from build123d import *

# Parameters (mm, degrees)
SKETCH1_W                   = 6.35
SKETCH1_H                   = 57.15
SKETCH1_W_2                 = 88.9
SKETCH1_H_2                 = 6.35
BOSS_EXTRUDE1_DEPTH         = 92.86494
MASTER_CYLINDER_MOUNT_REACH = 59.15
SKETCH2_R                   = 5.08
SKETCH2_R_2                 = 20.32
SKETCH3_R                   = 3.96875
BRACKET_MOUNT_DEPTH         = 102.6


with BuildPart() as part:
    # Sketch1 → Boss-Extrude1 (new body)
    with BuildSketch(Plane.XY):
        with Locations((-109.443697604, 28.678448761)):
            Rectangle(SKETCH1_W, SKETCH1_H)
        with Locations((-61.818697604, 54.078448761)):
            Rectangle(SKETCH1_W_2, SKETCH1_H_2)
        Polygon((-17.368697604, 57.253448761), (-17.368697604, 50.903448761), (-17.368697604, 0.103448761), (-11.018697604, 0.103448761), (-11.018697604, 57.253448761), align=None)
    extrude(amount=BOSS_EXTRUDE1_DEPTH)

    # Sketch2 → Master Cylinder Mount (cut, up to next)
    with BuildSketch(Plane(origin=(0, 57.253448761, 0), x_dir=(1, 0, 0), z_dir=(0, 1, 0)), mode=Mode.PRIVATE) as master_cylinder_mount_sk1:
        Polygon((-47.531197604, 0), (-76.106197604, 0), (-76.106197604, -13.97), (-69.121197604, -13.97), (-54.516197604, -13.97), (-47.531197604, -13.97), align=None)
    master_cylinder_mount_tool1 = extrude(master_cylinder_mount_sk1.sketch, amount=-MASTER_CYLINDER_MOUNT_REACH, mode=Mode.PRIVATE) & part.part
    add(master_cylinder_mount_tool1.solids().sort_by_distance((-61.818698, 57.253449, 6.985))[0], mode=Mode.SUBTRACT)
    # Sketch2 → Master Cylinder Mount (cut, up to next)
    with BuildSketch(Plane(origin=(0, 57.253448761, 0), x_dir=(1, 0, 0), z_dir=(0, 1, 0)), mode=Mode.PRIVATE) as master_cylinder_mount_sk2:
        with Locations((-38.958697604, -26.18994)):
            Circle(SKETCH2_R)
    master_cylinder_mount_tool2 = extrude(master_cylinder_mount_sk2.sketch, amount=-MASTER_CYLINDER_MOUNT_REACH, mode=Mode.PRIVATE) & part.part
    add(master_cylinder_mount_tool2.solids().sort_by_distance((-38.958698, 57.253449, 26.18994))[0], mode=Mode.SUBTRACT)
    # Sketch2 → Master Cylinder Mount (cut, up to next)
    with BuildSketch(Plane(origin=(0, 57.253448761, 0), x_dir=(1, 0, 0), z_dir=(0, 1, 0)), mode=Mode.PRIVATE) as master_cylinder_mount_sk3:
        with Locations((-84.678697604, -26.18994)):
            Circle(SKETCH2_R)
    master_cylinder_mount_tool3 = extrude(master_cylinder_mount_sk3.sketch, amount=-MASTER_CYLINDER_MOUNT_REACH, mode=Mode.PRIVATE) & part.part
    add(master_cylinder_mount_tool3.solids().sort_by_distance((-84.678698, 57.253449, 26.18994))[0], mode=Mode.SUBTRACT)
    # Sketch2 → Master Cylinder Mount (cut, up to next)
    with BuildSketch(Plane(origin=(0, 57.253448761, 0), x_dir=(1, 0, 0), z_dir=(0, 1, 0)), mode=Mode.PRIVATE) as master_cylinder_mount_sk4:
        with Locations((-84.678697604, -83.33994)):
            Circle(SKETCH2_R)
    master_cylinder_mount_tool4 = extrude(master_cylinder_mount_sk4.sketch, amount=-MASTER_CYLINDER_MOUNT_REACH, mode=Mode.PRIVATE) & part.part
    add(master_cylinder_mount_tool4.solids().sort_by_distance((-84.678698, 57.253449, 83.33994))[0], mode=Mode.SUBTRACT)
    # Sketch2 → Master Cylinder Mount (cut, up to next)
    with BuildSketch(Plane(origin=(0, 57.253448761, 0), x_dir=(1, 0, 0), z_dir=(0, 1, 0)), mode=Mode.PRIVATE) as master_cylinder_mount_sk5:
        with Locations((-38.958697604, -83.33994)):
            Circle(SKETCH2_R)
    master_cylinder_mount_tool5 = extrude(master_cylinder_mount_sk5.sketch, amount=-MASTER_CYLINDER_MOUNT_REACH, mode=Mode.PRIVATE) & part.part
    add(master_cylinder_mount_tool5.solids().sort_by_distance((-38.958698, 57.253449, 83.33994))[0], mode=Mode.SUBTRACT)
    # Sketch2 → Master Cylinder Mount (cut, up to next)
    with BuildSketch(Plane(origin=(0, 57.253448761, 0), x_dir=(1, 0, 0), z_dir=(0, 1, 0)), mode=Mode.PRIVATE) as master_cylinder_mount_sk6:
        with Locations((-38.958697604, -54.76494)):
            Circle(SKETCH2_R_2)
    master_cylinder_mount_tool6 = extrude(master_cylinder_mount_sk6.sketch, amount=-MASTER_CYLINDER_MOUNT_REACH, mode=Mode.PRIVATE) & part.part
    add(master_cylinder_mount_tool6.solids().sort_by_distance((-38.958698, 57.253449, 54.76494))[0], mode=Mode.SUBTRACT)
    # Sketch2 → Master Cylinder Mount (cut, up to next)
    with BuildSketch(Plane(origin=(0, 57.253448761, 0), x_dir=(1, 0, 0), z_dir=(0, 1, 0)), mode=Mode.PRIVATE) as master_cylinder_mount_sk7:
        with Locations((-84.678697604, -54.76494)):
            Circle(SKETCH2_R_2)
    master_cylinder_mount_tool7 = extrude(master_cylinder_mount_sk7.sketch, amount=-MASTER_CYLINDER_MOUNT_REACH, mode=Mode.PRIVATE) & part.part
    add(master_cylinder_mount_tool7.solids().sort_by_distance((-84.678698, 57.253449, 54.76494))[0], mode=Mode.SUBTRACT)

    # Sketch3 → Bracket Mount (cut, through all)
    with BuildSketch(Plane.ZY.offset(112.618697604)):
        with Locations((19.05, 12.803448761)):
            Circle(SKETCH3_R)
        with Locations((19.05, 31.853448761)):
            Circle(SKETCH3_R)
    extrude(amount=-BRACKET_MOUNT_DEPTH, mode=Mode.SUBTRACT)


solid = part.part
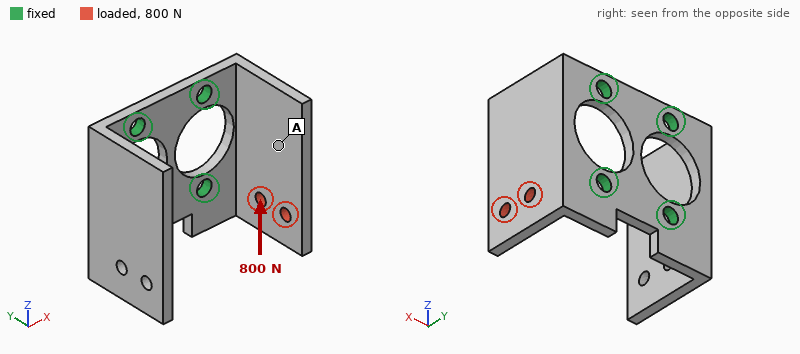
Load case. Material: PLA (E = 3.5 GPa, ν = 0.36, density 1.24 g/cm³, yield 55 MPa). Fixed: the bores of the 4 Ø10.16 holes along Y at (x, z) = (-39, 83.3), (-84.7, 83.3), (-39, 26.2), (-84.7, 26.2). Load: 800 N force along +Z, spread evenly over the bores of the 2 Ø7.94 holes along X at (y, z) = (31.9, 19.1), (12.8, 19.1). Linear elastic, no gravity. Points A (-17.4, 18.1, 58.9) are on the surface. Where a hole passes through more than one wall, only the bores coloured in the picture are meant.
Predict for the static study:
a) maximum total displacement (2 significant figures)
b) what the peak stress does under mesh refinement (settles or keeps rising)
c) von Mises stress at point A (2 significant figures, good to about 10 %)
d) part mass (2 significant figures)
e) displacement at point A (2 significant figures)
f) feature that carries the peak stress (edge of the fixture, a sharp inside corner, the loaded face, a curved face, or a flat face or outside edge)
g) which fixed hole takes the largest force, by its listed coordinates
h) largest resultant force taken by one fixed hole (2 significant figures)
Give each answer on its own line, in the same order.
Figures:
1.2 mm
keeps rising
3.9 MPa
120 g
0.62 mm
edge of the fixture
(-39, 26.2)
640 N
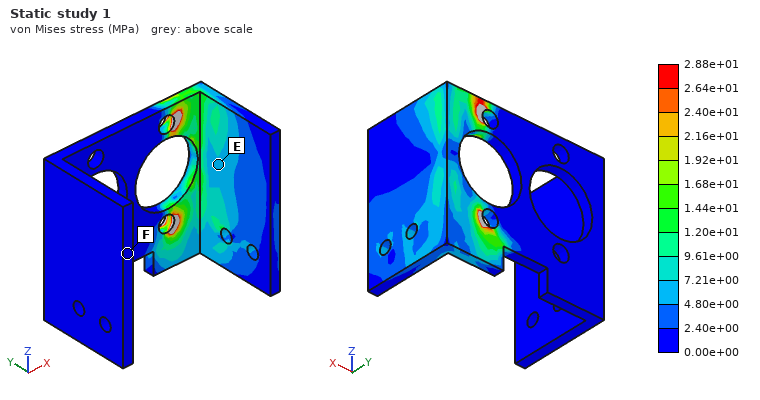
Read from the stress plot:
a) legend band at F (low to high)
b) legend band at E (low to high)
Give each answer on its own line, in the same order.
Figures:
0.00e+00 to 2.40e+00 MPa
4.80e+00 to 7.21e+00 MPa
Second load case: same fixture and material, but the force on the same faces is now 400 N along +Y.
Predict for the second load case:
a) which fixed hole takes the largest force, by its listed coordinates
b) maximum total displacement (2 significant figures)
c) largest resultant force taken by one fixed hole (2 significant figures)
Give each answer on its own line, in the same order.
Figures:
(-39, 26.2)
1.7 mm
420 N
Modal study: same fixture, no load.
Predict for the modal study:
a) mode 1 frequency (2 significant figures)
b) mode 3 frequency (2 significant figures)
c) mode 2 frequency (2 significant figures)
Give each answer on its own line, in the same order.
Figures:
310 Hz
670 Hz
310 Hz
